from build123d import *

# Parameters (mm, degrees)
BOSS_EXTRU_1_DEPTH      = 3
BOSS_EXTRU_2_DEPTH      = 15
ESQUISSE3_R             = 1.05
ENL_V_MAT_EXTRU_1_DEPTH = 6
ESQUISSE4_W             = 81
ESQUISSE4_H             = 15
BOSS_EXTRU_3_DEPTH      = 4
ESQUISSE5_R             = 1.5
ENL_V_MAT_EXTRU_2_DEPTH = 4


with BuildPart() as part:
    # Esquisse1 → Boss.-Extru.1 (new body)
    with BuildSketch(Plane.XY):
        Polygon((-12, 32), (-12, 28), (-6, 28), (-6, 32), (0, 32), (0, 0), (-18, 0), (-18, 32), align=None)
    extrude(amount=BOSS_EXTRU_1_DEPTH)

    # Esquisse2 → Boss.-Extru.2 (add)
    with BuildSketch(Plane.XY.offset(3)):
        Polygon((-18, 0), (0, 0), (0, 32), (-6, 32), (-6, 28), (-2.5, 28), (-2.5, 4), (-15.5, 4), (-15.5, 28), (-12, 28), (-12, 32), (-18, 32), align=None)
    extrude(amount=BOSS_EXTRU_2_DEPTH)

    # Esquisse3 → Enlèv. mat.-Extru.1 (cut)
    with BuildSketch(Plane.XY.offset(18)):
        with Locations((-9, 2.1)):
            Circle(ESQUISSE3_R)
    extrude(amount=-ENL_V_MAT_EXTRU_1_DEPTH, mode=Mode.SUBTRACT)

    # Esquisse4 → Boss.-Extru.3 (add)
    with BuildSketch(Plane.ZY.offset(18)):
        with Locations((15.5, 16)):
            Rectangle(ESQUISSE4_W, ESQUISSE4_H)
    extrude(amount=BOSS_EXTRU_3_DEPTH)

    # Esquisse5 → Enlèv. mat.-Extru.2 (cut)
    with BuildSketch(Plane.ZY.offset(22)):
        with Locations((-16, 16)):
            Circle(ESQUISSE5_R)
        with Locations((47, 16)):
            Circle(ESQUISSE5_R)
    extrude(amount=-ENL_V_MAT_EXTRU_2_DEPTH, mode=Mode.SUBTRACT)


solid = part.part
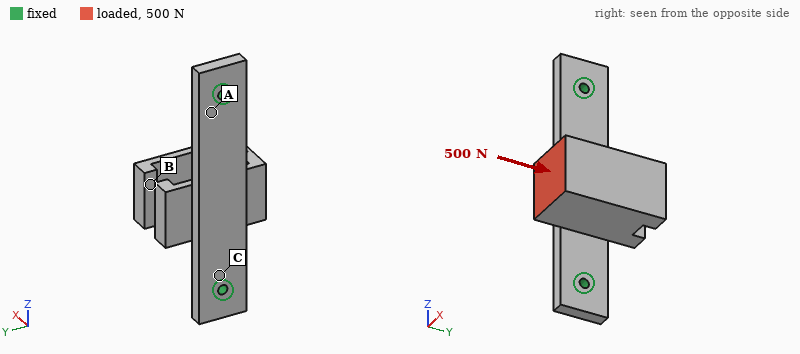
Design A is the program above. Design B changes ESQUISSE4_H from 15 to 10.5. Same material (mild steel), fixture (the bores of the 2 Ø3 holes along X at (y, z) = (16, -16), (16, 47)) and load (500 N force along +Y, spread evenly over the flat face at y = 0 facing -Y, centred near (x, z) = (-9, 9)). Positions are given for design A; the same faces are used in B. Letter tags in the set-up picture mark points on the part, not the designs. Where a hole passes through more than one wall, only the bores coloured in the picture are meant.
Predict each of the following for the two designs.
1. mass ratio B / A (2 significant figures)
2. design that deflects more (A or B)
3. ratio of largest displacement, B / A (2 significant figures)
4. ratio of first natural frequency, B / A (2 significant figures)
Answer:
0.85
B
1.6
0.80
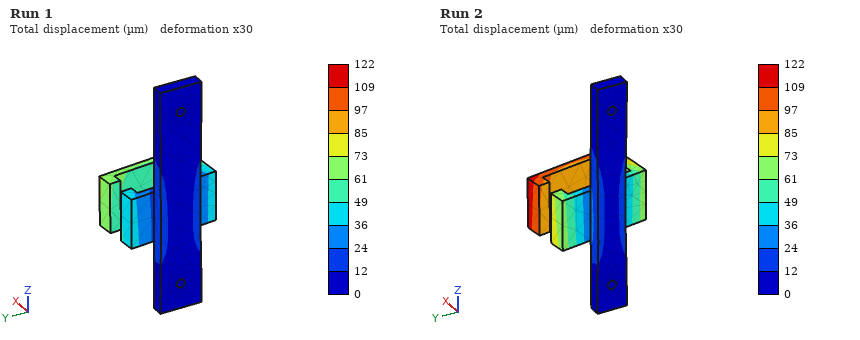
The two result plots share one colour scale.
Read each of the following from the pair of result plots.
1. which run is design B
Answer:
Run 2
